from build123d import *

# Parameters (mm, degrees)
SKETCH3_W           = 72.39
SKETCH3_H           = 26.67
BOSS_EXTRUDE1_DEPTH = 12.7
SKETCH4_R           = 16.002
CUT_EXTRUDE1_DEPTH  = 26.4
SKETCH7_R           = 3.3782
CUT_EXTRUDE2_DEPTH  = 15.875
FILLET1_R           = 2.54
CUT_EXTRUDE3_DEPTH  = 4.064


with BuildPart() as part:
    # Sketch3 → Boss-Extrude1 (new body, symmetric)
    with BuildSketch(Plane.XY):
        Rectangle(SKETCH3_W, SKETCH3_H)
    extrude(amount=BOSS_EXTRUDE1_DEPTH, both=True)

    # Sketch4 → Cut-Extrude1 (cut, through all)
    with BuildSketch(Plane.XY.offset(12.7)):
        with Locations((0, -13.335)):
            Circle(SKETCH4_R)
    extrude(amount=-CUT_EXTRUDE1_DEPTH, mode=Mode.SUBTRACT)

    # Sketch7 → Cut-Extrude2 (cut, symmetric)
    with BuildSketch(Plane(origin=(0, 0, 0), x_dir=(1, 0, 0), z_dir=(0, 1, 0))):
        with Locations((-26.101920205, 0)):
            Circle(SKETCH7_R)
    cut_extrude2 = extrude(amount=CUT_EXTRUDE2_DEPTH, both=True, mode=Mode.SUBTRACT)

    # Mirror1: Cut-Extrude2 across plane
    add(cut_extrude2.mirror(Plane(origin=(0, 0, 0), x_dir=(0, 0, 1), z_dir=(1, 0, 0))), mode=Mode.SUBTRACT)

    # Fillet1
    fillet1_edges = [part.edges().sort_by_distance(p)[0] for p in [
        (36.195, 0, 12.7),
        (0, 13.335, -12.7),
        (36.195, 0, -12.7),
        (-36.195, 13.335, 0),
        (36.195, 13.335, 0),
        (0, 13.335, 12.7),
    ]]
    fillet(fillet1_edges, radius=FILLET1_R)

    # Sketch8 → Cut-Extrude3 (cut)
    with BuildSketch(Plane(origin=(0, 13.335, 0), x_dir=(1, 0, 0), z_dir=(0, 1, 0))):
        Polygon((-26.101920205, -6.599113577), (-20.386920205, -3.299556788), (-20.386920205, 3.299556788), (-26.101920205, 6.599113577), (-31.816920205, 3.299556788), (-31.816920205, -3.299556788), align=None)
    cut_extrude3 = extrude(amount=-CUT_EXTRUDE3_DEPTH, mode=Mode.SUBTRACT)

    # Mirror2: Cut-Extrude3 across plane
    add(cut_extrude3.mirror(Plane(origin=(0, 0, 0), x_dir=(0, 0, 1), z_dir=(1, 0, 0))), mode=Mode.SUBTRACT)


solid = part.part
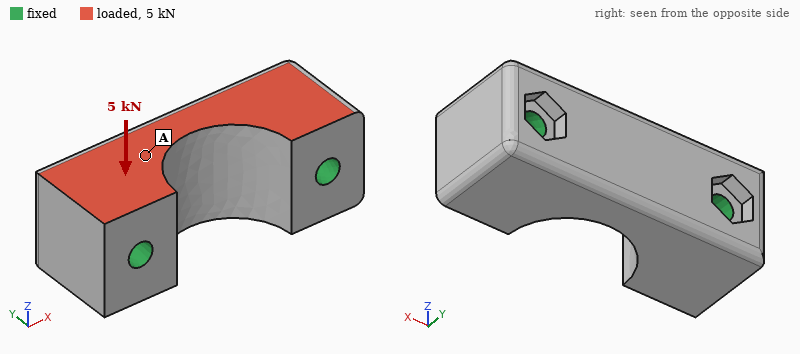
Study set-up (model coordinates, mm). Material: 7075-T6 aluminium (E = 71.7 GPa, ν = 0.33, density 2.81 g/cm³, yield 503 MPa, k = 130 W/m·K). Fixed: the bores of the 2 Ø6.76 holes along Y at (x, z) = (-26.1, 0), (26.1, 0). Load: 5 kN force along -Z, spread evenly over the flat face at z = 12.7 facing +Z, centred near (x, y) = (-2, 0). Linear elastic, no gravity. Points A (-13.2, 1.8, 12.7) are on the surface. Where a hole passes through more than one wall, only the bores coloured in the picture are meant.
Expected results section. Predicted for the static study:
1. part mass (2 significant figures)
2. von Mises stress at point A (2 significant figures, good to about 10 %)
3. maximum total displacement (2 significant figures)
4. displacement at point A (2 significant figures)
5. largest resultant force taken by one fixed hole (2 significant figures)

100 g
3.4 MPa
3.5 µm
2.5 µm
2.6 kN
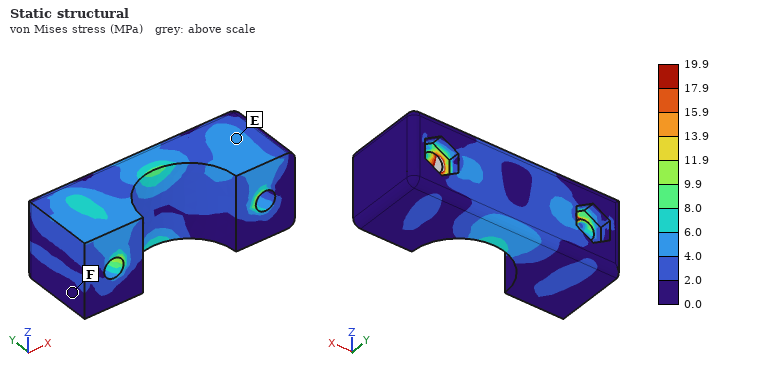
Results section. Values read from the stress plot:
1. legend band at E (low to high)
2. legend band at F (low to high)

4.0 to 6.0 MPa
0.0 to 2.0 MPa
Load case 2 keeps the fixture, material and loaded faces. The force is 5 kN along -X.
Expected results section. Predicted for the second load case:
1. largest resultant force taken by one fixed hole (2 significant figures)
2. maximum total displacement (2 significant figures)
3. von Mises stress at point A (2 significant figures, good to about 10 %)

2.7 kN
4.7 µm
8.4 MPa
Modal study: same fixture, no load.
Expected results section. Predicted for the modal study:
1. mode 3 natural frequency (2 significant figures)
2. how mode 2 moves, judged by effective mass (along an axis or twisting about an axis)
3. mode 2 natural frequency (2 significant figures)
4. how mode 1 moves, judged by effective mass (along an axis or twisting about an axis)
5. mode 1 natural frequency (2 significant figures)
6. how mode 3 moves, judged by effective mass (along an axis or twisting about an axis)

33 kHz
along Y
26 kHz
along Z
20 kHz
twisting about X
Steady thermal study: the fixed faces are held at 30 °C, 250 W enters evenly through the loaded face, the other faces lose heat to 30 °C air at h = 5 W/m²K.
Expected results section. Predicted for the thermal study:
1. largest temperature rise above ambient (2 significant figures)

28 K
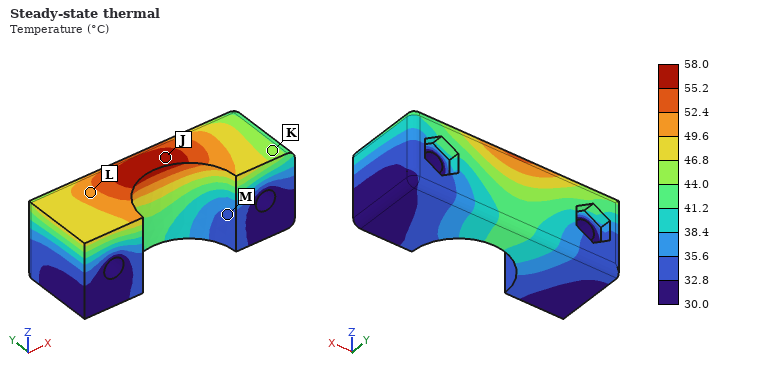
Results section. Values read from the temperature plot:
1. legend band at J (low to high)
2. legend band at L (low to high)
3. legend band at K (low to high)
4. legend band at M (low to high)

55.2 to 58.0 °C
49.6 to 52.4 °C
44.0 to 46.8 °C
32.8 to 35.6 °C
